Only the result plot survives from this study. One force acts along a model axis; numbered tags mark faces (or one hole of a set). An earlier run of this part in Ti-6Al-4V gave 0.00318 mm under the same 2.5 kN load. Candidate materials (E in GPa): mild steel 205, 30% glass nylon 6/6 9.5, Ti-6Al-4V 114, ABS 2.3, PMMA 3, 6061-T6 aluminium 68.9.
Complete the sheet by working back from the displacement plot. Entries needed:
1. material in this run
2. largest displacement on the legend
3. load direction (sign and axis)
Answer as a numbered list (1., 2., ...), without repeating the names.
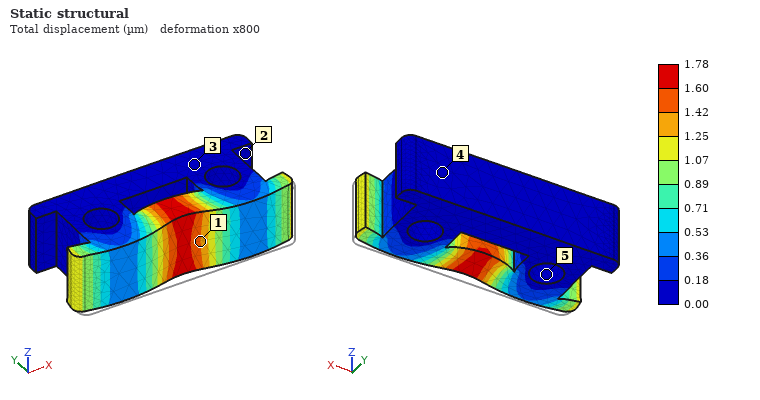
1. mild steel
2. 1.78 µm
3. +Y
